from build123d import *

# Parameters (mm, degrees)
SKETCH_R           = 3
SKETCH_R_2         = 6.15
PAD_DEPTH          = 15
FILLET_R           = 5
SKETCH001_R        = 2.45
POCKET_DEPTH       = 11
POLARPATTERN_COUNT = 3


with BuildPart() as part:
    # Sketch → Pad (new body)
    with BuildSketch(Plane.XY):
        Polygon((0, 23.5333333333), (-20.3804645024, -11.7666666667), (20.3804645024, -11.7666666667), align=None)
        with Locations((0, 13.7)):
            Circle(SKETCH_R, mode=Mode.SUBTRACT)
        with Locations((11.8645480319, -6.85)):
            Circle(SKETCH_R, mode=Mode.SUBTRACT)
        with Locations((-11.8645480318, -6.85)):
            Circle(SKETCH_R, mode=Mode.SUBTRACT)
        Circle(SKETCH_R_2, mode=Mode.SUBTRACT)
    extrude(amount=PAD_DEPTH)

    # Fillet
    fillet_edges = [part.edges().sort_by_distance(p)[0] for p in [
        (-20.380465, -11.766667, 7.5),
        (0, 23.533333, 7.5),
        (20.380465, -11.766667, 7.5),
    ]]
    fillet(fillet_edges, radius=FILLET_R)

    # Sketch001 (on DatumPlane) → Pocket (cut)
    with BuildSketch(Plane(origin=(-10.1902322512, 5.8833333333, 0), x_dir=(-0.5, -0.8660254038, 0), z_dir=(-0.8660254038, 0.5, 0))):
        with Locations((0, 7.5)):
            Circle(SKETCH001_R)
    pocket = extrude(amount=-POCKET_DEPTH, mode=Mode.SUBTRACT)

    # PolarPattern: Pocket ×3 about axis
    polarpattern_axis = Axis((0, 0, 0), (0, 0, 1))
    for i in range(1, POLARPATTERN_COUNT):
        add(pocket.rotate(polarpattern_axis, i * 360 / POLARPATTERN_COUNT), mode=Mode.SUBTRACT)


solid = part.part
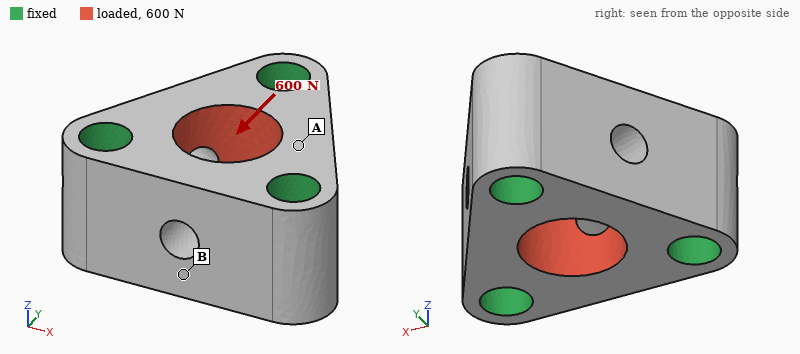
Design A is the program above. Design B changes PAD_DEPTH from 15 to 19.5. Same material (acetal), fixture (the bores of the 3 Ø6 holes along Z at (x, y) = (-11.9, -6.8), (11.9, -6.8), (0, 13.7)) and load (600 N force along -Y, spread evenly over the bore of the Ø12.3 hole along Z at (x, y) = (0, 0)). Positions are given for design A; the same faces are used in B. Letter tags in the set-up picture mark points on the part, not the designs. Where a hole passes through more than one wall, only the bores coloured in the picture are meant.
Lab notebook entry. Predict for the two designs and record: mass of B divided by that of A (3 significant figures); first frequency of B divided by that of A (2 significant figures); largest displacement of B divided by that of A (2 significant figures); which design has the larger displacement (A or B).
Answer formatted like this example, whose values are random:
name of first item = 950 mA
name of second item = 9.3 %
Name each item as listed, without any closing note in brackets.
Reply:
mass of B divided by that of A = 1.31
first frequency of B divided by that of A = 1.00
largest displacement of B divided by that of A = 0.77
which design has the larger displacement = A
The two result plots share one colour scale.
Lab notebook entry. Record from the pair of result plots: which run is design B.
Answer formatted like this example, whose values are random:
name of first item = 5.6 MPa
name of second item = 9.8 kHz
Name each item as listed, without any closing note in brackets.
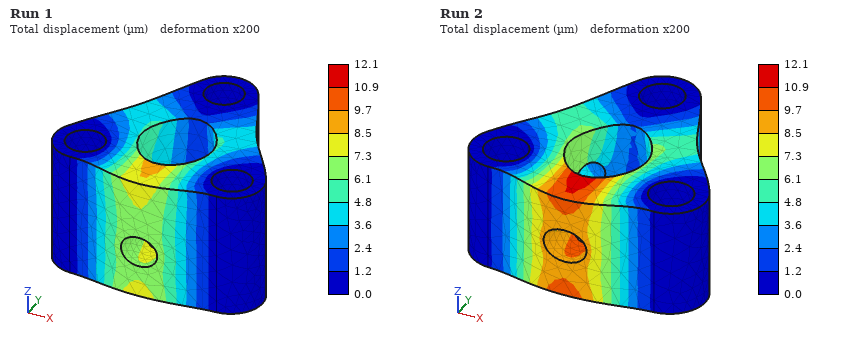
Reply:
which run is design B = Run 1
